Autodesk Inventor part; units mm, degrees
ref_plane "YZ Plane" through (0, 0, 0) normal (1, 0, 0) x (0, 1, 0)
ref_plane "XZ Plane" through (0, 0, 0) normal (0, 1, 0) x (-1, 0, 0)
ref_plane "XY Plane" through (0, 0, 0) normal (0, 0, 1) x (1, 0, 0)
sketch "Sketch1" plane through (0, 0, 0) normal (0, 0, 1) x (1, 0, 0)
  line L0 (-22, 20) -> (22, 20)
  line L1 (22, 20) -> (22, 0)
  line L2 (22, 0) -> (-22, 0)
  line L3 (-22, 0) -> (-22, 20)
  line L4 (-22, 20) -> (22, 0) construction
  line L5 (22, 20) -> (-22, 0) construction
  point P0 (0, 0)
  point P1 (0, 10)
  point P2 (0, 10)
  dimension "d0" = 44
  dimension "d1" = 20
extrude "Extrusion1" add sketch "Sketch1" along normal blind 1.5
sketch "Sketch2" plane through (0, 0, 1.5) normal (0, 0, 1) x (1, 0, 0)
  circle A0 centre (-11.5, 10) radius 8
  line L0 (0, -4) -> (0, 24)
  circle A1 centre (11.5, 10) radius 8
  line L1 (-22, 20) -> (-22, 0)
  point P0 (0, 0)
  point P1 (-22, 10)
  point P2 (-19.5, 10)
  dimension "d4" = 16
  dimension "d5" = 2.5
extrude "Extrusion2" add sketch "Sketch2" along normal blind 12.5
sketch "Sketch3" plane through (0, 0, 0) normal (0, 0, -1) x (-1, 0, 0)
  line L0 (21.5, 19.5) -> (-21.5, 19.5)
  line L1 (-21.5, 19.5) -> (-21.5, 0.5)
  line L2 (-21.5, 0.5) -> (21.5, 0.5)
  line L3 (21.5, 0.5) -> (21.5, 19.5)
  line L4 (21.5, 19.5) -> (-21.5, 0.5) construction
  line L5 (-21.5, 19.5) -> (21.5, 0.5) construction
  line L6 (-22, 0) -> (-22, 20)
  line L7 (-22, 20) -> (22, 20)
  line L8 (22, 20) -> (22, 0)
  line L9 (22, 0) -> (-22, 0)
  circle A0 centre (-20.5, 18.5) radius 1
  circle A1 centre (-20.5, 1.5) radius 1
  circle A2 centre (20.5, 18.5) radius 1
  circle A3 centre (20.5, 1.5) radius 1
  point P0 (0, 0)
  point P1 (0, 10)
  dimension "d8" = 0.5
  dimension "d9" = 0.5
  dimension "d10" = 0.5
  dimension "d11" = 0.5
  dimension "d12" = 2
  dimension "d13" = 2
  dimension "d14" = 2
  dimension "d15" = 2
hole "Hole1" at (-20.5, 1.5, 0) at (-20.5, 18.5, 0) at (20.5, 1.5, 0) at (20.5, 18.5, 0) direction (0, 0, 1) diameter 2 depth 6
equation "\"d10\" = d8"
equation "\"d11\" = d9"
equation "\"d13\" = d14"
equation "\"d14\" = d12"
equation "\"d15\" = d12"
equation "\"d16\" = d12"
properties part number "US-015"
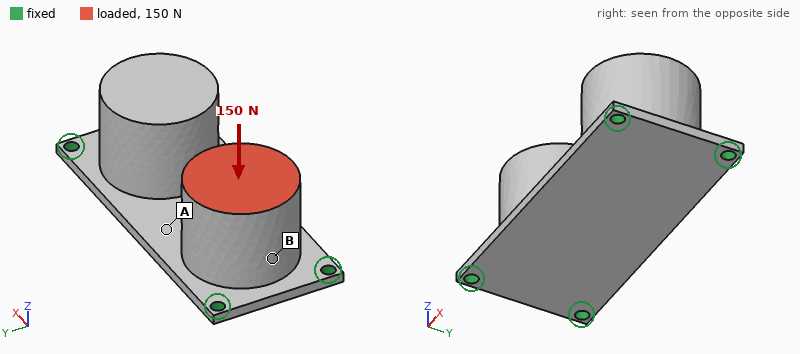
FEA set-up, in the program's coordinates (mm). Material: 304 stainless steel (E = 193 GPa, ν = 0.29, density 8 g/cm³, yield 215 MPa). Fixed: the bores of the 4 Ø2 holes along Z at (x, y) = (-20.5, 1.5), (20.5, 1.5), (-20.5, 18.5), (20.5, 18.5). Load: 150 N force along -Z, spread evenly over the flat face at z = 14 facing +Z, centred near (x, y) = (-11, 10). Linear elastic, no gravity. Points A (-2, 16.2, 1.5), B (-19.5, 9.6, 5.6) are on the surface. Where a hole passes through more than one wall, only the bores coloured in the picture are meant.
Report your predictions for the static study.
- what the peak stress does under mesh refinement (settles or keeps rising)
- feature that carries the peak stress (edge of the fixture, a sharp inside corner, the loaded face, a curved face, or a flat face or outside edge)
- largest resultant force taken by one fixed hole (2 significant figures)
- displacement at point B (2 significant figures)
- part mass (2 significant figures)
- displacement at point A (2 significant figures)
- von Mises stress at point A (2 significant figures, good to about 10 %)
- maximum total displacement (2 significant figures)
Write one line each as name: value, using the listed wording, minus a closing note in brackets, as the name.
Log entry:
what the peak stress does under mesh refinement: keeps rising
feature that carries the peak stress: edge of the fixture
largest resultant force taken by one fixed hole: 63 N
displacement at point B: 5.9 µm
part mass: 51 g
displacement at point A: 20 µm
von Mises stress at point A: 34 MPa
maximum total displacement: 26 µm
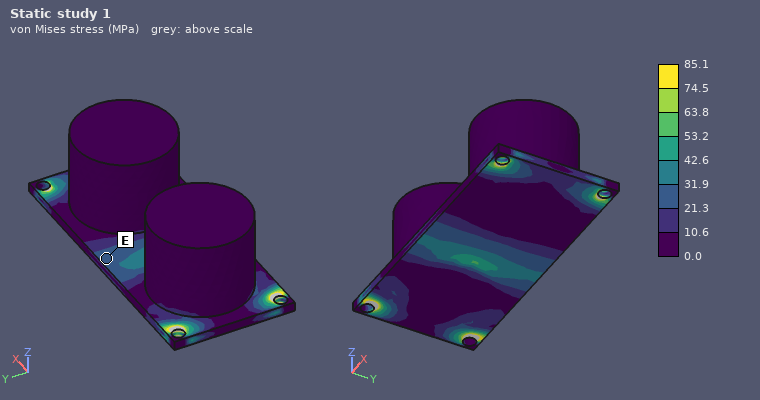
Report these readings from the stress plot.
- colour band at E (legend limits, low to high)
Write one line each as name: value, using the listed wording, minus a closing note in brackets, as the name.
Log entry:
colour band at E: 21.3 to 31.9 MPa
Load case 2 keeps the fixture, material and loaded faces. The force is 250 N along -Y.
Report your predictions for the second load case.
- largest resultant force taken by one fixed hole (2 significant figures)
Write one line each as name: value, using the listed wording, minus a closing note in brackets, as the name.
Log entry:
largest resultant force taken by one fixed hole: 250 N
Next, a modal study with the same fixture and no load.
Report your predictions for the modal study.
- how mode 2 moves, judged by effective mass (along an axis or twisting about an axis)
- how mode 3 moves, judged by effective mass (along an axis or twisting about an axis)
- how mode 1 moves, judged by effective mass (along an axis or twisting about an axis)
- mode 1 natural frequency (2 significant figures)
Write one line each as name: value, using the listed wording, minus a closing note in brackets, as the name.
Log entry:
how mode 2 moves, judged by effective mass: along Y
how mode 3 moves, judged by effective mass: twisting about Z
how mode 1 moves, judged by effective mass: along Z
mode 1 natural frequency: 1900 Hz
